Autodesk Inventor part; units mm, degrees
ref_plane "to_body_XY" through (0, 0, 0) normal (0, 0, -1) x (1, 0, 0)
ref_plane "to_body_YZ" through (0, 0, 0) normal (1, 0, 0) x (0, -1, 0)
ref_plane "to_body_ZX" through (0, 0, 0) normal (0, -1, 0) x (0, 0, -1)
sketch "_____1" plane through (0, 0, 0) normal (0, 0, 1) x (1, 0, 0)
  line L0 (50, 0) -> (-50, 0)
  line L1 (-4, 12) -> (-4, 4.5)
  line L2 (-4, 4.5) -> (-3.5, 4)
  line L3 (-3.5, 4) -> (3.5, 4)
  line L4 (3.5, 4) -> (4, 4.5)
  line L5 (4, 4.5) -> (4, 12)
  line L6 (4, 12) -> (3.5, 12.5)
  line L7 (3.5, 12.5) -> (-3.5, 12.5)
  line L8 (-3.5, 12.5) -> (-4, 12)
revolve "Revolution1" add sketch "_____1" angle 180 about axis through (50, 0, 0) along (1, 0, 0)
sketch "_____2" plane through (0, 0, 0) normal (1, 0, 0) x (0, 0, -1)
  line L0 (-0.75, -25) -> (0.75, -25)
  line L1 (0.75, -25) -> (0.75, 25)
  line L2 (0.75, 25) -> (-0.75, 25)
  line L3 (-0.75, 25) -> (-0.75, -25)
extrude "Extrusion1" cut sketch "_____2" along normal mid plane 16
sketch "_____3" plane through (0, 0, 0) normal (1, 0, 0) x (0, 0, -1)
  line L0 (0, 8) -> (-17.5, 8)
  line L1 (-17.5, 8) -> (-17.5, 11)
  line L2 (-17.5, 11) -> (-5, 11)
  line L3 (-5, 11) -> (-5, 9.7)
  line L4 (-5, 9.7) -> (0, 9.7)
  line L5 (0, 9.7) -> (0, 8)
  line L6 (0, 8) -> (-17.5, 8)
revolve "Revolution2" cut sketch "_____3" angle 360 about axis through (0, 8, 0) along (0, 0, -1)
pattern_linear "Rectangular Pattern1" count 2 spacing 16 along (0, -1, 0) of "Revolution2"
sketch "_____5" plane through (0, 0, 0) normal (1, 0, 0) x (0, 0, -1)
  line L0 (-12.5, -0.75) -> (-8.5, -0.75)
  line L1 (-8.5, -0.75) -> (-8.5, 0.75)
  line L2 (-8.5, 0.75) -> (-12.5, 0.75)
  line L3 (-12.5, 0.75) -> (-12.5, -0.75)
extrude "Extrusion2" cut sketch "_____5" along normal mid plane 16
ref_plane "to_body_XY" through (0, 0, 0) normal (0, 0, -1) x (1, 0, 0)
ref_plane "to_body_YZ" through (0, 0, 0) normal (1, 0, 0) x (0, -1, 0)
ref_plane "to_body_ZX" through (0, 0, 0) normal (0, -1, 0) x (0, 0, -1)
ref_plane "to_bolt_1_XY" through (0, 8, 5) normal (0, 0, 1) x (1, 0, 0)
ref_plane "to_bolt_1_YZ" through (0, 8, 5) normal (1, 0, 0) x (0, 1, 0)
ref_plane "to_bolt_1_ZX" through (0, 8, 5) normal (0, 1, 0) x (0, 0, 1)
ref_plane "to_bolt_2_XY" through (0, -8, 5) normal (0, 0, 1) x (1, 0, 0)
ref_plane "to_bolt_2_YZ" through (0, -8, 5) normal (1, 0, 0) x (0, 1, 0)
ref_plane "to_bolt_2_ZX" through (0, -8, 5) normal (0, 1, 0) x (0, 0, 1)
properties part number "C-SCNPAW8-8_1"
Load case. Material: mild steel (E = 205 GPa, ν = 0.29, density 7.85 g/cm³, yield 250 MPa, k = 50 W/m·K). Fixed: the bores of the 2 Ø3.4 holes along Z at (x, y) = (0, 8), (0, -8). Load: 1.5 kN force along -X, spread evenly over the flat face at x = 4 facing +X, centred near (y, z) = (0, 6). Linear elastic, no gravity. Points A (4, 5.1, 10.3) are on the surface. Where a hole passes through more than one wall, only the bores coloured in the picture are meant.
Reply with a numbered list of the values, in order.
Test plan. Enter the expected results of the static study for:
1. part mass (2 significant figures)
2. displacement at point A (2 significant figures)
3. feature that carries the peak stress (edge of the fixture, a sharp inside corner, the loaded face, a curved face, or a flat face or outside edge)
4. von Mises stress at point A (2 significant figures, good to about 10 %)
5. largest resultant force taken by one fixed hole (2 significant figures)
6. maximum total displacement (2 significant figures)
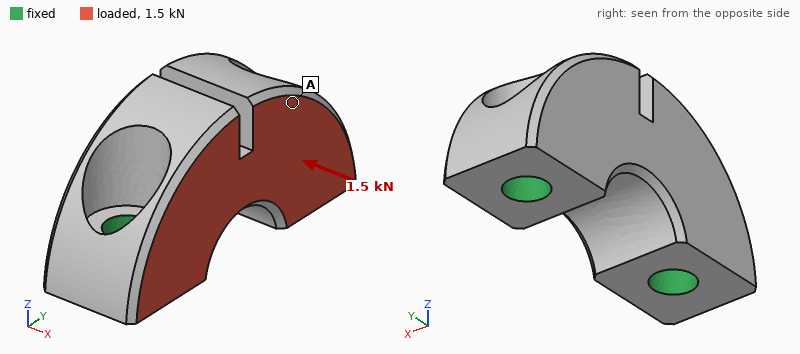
1. 10 g
2. 4.5 µm
3. edge of the fixture
4. 20 MPa
5. 750 N
6. 5.1 µm
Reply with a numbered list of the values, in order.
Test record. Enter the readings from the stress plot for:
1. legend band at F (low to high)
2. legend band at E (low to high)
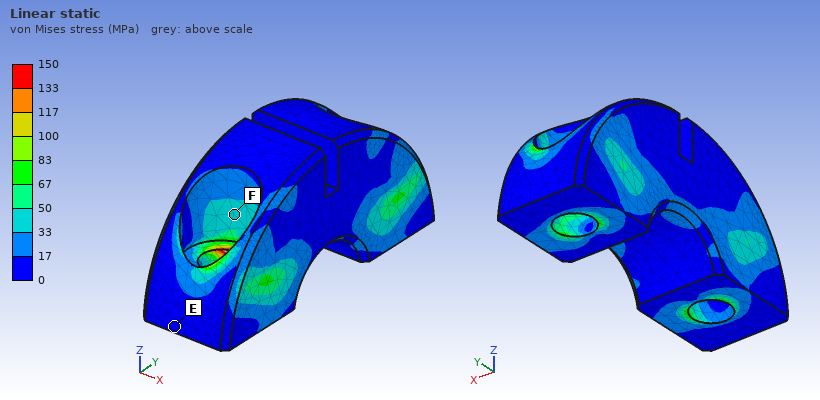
1. 33 to 50 MPa
2. 0 to 17 MPa
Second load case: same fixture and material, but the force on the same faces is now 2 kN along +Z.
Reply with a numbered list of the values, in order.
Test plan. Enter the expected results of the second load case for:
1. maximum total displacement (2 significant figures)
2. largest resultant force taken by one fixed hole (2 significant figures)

1. 6.7 µm
2. 1.0 kN
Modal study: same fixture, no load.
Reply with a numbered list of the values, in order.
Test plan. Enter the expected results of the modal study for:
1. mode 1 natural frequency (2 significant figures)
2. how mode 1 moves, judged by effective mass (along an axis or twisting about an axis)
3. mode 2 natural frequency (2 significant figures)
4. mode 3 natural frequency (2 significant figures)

1. 32 kHz
2. along X
3. 62 kHz
4. 63 kHz
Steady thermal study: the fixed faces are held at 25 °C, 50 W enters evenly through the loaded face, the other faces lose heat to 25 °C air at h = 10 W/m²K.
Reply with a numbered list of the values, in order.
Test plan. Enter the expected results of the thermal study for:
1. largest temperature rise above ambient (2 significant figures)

1. 63 K
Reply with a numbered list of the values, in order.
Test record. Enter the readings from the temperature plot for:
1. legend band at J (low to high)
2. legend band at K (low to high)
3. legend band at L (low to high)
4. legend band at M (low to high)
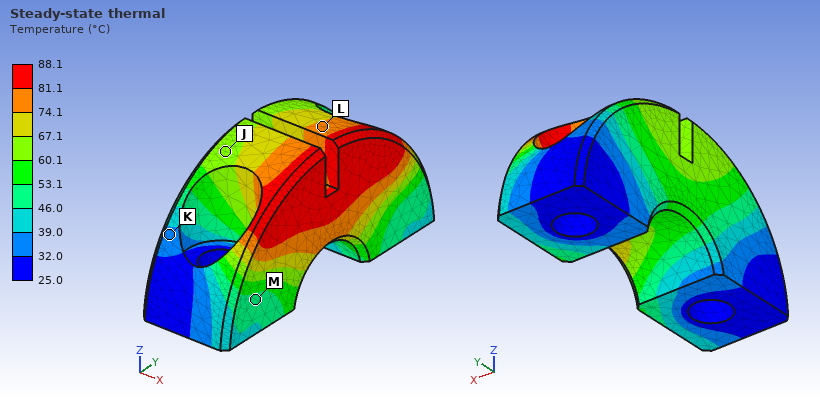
1. 60.1 to 67.1 °C
2. 32.0 to 39.0 °C
3. 74.1 to 81.1 °C
4. 46.0 to 53.1 °C
